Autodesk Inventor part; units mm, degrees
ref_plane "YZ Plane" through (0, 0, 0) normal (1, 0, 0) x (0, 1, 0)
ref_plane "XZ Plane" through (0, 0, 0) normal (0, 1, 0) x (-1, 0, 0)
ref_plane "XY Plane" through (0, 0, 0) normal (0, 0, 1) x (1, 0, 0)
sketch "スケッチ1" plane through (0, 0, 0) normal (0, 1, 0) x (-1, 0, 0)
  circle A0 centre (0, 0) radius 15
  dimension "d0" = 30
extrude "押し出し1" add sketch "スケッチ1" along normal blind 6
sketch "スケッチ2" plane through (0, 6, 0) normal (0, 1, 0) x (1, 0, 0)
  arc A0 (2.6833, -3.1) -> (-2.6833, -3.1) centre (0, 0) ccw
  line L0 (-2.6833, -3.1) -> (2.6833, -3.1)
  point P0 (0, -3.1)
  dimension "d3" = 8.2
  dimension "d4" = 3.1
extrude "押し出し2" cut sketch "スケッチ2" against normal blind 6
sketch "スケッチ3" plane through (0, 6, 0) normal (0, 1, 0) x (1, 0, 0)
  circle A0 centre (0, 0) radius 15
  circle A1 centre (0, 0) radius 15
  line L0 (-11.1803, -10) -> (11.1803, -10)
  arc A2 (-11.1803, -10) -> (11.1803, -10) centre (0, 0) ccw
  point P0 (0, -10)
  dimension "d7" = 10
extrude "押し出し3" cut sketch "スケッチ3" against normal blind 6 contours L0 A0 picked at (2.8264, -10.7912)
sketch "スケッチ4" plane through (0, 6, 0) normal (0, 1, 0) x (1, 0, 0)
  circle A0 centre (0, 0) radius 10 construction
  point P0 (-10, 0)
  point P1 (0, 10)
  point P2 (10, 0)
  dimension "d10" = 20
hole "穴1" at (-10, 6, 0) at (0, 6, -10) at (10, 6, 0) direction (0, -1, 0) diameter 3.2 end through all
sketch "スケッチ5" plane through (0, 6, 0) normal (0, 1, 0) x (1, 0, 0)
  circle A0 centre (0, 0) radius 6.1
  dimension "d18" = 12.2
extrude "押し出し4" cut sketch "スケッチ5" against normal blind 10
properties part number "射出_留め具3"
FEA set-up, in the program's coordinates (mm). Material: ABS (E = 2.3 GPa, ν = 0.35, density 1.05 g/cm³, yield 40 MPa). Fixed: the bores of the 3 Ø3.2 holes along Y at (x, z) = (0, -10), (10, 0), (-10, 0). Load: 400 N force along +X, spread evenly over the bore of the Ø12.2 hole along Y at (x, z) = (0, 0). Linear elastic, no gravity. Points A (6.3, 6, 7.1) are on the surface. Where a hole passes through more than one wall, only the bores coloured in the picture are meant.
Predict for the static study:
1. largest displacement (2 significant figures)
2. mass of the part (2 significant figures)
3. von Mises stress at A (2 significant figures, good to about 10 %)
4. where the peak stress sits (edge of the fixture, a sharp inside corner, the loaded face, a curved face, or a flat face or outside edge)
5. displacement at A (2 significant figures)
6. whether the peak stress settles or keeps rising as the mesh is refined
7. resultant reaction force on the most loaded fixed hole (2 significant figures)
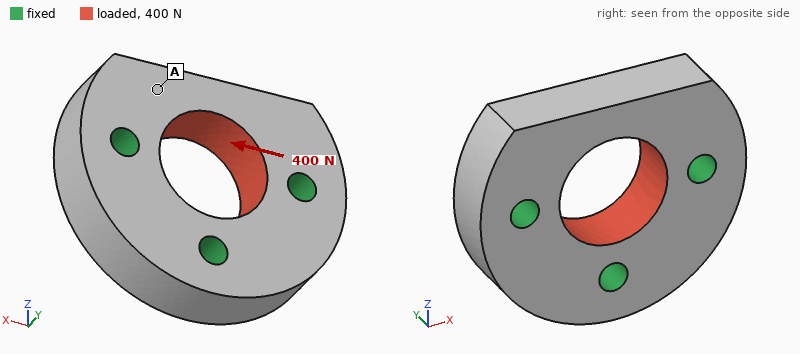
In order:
23 µm
3.1 g
1.6 MPa
edge of the fixture
18 µm
keeps rising
160 N
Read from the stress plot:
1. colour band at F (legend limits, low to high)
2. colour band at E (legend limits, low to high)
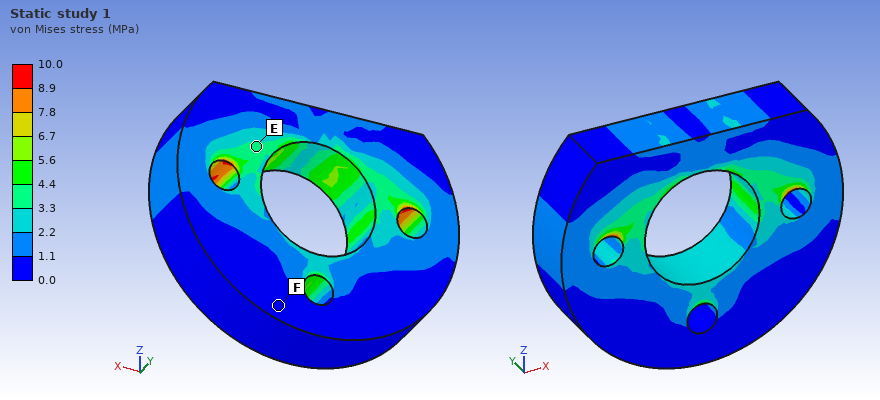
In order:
0.0 to 1.1 MPa
3.3 to 4.4 MPa
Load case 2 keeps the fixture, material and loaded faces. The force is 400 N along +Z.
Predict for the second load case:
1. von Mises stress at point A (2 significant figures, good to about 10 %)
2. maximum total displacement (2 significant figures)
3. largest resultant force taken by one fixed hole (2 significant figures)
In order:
2.2 MPa
27 µm
150 N
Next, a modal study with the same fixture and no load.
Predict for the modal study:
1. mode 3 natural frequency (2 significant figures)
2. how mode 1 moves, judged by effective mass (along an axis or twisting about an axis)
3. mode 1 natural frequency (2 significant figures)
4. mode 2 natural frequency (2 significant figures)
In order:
15 kHz
along Y
9700 Hz
14 kHz
